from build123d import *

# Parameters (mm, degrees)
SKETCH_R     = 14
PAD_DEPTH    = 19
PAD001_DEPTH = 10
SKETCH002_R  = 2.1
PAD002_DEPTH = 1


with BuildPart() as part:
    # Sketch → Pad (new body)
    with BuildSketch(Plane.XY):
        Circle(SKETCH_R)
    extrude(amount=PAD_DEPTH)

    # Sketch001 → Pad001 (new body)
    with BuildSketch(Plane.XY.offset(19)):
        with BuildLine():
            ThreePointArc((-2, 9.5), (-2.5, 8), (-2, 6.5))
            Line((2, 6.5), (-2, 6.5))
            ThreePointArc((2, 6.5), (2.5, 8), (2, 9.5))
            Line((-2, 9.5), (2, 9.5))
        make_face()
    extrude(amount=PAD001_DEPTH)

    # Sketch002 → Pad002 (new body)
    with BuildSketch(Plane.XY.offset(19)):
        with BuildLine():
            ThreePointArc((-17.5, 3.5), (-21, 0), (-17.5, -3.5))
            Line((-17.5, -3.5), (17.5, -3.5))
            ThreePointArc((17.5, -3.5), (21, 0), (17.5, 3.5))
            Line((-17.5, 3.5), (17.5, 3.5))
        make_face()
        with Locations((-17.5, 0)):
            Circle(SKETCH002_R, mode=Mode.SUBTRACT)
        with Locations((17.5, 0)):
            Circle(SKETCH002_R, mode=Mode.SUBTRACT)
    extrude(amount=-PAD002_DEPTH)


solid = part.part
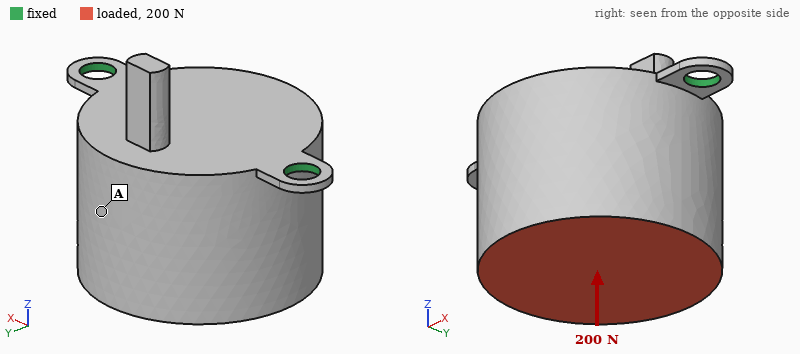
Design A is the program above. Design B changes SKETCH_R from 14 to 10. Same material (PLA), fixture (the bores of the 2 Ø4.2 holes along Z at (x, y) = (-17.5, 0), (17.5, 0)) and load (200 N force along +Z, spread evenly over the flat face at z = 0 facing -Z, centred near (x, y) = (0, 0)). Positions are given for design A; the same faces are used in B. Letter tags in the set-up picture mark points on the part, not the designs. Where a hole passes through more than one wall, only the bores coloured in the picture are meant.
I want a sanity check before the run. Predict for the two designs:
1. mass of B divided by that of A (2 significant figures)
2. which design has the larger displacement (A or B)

0.52
B
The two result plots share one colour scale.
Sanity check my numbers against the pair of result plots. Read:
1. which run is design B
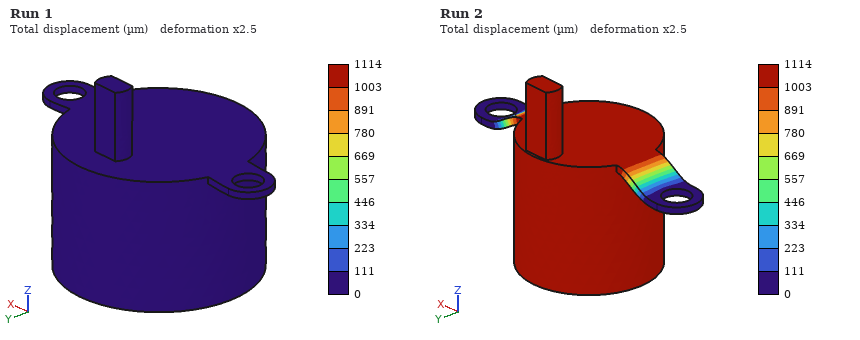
Run 2
